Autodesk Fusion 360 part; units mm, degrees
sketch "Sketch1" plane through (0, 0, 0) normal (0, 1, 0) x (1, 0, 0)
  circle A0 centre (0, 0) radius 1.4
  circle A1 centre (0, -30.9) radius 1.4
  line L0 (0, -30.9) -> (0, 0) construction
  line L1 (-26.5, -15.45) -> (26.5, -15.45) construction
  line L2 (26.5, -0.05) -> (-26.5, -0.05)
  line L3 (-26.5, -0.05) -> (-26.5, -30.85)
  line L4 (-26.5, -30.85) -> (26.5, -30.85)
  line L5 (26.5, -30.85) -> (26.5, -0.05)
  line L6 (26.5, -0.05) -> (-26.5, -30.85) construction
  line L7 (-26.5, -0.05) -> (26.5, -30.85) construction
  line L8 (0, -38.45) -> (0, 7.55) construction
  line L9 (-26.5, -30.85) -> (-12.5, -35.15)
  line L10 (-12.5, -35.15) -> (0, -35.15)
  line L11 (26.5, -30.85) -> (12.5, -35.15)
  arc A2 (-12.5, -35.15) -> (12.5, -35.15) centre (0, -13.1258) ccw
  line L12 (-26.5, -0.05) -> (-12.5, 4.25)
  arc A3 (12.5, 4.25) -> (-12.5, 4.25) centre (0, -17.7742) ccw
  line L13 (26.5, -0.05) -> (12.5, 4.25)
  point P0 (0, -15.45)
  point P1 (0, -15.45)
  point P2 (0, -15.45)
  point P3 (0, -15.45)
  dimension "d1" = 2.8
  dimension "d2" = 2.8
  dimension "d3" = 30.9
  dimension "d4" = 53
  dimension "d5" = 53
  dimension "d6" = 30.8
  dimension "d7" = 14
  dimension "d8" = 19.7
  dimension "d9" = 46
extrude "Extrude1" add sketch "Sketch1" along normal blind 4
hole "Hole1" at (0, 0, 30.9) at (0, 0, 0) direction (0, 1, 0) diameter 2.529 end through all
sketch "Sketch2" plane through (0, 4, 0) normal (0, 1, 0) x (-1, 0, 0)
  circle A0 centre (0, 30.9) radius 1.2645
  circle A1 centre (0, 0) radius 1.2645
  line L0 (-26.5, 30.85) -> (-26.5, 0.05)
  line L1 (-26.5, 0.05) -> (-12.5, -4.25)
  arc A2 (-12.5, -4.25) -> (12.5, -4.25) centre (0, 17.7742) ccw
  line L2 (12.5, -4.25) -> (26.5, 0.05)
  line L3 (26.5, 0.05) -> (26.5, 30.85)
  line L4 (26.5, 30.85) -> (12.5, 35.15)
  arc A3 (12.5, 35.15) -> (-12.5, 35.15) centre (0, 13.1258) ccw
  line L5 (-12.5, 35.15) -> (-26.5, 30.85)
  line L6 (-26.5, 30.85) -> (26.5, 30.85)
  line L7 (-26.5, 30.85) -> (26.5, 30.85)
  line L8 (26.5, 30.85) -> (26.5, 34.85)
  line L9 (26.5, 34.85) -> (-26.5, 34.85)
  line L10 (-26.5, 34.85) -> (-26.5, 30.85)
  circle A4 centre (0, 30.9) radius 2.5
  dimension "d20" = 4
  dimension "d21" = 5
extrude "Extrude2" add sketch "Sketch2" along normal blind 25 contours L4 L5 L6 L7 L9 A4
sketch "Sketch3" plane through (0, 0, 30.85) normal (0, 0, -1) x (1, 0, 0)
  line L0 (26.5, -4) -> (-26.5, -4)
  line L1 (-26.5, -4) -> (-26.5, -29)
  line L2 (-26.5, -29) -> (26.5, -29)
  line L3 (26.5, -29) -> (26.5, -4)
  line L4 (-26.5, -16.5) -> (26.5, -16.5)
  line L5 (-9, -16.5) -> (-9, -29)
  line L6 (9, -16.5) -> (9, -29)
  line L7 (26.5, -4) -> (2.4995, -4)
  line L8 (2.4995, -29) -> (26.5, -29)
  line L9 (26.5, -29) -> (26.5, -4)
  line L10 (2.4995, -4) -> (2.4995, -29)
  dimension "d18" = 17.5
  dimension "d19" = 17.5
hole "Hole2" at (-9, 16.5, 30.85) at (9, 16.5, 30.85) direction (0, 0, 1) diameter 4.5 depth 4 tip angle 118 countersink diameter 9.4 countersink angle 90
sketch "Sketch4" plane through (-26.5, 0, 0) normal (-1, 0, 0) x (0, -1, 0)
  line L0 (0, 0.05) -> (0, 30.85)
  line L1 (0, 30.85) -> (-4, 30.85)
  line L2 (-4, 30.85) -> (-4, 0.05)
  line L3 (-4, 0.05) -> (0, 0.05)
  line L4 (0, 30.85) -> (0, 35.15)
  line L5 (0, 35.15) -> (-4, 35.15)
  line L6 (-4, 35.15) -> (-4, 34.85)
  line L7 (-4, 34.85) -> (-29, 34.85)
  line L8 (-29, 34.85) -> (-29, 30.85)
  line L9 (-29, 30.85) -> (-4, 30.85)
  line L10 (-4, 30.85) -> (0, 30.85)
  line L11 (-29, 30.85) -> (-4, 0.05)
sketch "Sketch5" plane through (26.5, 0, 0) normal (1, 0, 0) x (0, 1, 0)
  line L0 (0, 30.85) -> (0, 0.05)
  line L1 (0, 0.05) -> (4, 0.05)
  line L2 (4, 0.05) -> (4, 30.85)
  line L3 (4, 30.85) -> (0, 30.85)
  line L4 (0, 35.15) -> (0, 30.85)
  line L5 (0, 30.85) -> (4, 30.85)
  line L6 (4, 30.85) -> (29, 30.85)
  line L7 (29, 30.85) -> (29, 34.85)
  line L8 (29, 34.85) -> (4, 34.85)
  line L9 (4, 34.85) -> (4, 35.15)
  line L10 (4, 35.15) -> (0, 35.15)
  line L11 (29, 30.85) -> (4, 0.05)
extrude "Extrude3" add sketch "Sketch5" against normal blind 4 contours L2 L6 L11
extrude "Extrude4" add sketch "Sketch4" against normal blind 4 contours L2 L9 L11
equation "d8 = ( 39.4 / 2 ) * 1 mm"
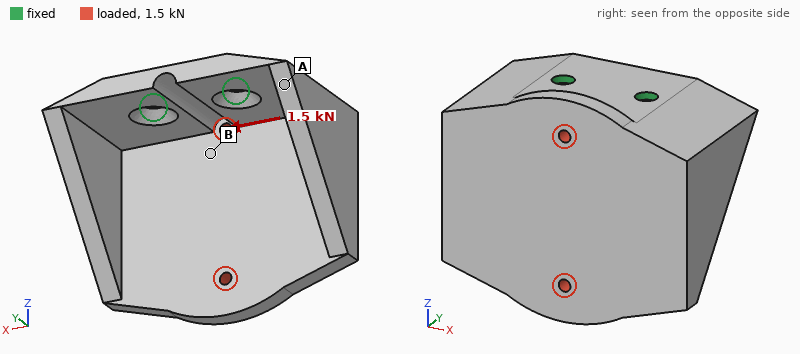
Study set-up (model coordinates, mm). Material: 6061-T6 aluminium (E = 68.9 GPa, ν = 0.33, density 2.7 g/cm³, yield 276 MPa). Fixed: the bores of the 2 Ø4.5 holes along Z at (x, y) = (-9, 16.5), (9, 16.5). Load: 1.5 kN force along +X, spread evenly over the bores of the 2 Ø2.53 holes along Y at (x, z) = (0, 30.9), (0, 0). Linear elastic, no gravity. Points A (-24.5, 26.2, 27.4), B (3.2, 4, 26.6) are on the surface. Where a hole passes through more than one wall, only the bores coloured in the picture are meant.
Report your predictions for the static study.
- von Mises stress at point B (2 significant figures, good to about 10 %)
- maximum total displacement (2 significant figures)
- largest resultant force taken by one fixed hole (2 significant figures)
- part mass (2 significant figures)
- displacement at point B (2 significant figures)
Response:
49 MPa
0.35 mm
1.8 kN
40 g
0.068 mm
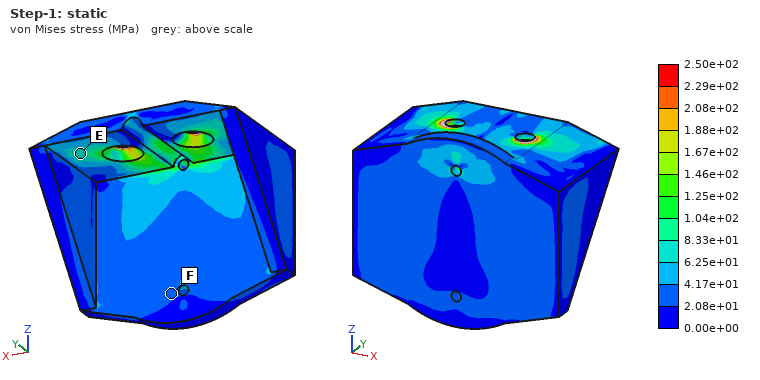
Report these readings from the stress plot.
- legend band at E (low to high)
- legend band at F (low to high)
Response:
6.25e+01 to 8.33e+01 MPa
2.08e+01 to 4.17e+01 MPa
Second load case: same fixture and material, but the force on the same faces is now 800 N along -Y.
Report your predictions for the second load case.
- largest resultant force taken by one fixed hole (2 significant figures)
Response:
400 N
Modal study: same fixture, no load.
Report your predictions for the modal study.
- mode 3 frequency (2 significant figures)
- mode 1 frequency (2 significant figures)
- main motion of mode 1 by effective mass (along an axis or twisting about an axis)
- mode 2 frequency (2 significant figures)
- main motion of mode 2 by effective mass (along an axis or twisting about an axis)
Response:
4600 Hz
1300 Hz
along Y
2000 Hz
along X
